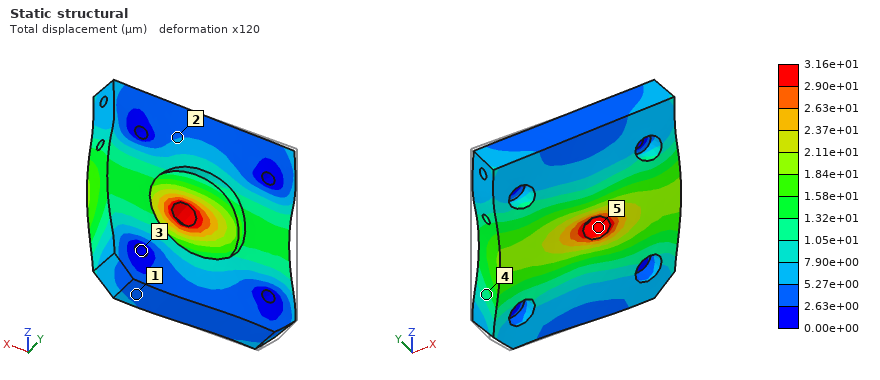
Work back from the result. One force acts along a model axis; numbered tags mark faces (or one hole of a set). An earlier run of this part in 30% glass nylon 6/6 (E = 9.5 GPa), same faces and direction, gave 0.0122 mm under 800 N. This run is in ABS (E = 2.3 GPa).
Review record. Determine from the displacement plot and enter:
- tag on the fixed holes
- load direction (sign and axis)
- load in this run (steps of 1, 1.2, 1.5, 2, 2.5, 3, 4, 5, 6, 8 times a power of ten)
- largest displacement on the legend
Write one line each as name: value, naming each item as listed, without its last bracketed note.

tag on the fixed holes: 3
load direction: +X
load in this run: 500 N
largest displacement on the legend: 3.16e+01 µm
